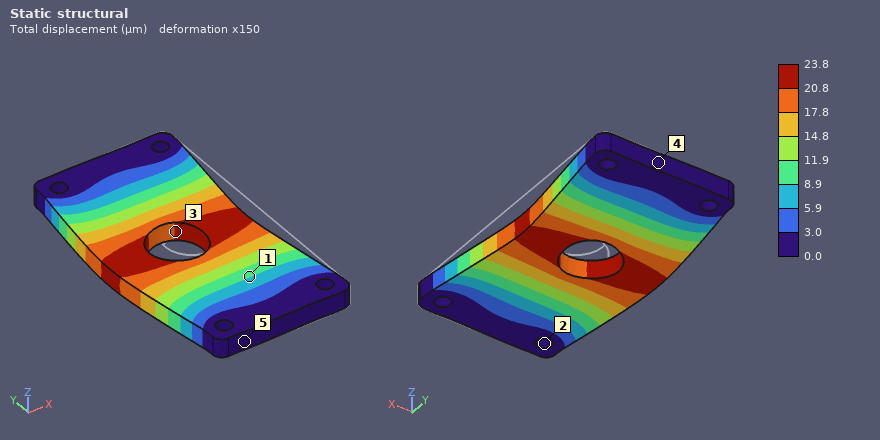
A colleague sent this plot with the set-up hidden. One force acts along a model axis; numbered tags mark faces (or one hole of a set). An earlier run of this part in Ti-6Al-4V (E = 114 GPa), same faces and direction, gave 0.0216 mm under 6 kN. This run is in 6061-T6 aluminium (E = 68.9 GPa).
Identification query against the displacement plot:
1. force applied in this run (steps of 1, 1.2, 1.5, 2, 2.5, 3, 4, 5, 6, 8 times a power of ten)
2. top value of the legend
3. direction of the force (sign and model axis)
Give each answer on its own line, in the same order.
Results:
4 kN
23.8 µm
-X
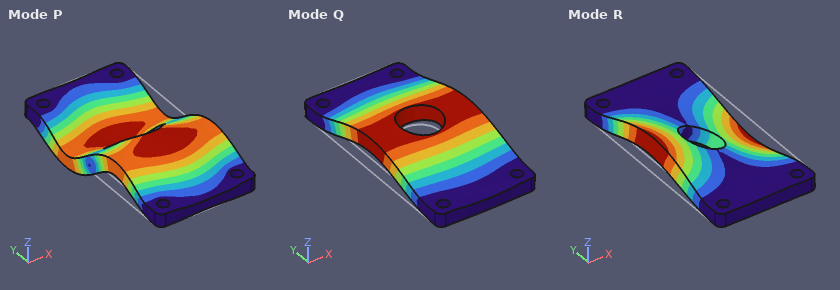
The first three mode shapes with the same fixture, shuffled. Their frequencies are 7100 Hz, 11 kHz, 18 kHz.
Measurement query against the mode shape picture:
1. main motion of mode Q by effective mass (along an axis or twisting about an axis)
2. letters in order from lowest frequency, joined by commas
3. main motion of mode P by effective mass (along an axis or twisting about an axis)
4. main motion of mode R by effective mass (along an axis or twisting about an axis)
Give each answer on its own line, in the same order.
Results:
along Z
Q, R, P
twisting about X
twisting about Y
